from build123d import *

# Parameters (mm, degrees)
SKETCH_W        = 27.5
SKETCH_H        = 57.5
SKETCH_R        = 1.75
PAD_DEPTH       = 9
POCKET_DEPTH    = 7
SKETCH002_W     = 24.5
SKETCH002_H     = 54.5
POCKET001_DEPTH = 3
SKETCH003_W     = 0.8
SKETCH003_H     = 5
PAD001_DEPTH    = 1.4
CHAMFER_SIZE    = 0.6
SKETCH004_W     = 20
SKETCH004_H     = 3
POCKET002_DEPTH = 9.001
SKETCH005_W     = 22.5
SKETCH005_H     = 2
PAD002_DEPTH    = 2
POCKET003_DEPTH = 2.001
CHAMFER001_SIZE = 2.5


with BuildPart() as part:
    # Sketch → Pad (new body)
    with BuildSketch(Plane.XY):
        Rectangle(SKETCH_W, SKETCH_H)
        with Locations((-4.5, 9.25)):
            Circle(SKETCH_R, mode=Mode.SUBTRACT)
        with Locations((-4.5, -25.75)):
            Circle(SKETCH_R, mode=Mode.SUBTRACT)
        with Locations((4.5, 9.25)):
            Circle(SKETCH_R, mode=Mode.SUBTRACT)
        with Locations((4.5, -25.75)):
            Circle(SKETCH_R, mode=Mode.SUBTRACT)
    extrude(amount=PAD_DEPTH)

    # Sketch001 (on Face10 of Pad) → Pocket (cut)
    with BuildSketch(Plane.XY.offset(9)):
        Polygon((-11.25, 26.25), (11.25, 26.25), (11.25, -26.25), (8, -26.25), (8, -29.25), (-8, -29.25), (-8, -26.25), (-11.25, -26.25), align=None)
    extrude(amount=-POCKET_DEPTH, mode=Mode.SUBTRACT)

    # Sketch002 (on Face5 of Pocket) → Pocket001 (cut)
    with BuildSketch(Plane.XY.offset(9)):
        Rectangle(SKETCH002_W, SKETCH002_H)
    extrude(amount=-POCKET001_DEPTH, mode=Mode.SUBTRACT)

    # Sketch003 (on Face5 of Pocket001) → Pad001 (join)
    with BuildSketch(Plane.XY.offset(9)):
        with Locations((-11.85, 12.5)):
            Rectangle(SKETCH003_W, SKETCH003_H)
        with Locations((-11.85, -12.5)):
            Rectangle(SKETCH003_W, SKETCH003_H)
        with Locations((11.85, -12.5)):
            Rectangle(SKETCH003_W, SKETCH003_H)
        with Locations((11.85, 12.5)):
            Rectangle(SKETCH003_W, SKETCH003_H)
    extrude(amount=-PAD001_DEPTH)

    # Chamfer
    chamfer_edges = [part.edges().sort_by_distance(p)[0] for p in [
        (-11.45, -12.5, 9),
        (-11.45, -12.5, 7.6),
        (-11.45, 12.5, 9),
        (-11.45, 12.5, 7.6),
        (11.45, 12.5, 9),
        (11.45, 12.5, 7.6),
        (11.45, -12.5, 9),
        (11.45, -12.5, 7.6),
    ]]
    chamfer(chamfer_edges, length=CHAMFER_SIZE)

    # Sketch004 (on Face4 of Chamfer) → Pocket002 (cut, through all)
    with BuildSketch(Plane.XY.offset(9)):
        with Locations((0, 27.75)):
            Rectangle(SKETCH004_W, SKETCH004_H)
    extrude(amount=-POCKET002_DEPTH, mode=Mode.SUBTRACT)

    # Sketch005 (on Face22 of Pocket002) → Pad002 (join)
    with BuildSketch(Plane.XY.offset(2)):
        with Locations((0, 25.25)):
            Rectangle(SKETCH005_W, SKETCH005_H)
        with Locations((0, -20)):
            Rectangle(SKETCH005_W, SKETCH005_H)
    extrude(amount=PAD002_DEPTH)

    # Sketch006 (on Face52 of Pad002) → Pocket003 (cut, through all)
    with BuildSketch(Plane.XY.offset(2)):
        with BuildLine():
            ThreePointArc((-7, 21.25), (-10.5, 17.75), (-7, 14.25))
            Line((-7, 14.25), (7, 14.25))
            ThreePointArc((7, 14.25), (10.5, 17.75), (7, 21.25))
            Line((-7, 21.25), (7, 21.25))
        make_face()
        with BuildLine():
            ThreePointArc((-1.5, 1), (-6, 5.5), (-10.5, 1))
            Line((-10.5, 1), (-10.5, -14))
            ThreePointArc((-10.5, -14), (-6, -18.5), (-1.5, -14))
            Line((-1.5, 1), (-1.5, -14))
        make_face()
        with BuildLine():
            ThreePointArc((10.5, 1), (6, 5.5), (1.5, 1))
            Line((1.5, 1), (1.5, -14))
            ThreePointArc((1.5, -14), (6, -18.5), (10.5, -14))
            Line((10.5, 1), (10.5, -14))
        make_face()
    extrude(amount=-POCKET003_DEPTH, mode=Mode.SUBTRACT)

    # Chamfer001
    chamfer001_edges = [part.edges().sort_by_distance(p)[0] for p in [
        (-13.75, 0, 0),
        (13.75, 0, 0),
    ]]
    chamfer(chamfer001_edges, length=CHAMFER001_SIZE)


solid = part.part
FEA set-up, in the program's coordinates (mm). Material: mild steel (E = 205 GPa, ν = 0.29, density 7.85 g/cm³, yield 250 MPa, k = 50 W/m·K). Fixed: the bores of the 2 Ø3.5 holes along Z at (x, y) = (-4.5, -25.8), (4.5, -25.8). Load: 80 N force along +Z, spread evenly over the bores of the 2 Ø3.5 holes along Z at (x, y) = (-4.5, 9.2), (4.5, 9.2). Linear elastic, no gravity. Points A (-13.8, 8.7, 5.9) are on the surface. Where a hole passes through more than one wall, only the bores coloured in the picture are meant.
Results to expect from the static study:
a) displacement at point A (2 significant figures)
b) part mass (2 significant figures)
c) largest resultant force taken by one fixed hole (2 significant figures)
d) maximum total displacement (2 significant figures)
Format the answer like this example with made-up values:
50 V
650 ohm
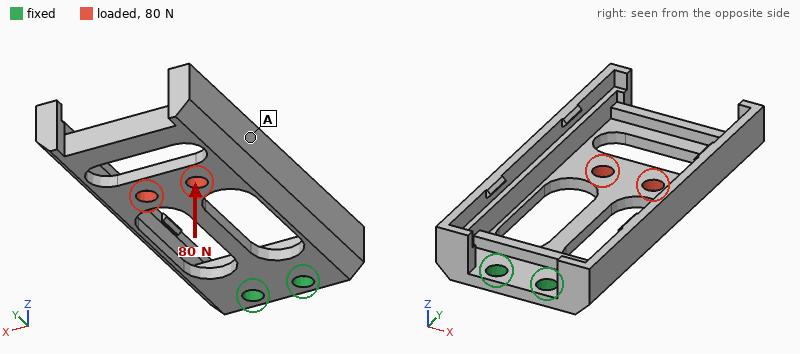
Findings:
0.086 mm
28 g
52 N
0.14 mm
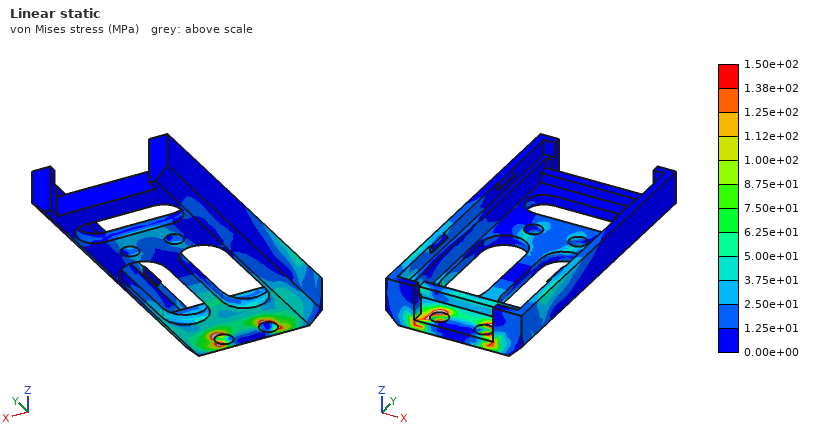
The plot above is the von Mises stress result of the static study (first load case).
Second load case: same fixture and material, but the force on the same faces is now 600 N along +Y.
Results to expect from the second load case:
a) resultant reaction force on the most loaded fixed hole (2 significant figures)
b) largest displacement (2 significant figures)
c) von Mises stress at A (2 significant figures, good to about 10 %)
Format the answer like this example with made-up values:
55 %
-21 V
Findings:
300 N
25 µm
5.1 MPa
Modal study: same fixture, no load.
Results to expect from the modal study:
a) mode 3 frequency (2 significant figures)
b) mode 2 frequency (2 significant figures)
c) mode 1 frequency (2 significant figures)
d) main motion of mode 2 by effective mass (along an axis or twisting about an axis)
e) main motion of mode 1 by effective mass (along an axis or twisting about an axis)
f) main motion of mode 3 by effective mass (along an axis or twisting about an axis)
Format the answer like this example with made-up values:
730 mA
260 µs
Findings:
2300 Hz
1600 Hz
1000 Hz
along X
along Z
along X
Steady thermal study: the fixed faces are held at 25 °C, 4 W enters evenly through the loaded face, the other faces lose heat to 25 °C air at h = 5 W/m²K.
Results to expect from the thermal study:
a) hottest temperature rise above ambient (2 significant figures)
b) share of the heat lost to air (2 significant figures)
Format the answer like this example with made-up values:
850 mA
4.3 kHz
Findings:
65 K
18 %
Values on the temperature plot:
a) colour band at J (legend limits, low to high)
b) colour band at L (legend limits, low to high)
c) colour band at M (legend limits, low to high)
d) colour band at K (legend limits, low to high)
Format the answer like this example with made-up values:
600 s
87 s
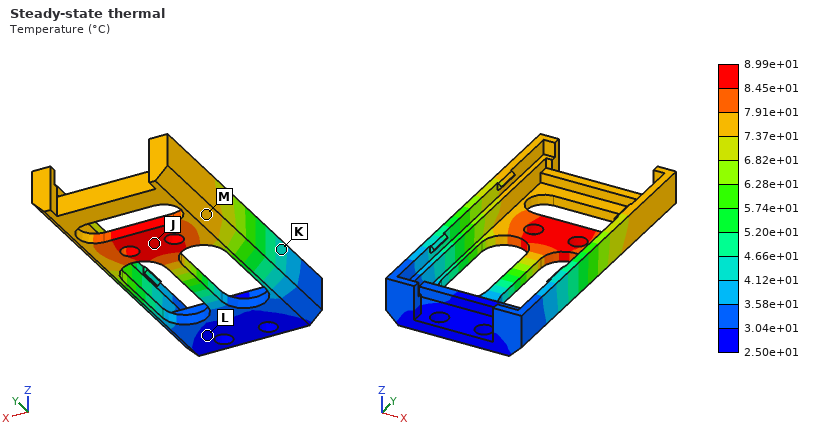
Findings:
8.45e+01 to 8.99e+01 °C
2.50e+01 to 3.04e+01 °C
7.37e+01 to 7.91e+01 °C
4.12e+01 to 4.66e+01 °C
